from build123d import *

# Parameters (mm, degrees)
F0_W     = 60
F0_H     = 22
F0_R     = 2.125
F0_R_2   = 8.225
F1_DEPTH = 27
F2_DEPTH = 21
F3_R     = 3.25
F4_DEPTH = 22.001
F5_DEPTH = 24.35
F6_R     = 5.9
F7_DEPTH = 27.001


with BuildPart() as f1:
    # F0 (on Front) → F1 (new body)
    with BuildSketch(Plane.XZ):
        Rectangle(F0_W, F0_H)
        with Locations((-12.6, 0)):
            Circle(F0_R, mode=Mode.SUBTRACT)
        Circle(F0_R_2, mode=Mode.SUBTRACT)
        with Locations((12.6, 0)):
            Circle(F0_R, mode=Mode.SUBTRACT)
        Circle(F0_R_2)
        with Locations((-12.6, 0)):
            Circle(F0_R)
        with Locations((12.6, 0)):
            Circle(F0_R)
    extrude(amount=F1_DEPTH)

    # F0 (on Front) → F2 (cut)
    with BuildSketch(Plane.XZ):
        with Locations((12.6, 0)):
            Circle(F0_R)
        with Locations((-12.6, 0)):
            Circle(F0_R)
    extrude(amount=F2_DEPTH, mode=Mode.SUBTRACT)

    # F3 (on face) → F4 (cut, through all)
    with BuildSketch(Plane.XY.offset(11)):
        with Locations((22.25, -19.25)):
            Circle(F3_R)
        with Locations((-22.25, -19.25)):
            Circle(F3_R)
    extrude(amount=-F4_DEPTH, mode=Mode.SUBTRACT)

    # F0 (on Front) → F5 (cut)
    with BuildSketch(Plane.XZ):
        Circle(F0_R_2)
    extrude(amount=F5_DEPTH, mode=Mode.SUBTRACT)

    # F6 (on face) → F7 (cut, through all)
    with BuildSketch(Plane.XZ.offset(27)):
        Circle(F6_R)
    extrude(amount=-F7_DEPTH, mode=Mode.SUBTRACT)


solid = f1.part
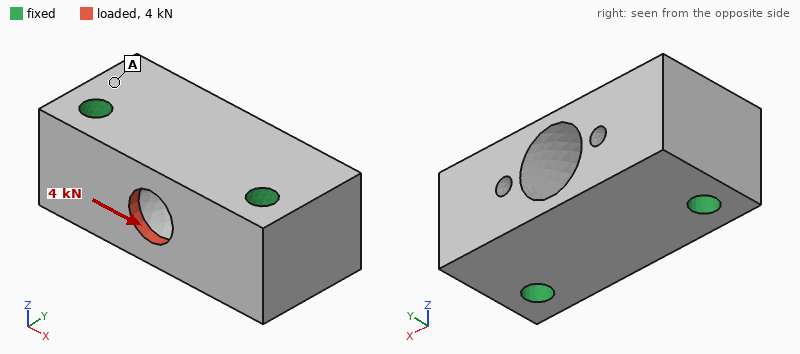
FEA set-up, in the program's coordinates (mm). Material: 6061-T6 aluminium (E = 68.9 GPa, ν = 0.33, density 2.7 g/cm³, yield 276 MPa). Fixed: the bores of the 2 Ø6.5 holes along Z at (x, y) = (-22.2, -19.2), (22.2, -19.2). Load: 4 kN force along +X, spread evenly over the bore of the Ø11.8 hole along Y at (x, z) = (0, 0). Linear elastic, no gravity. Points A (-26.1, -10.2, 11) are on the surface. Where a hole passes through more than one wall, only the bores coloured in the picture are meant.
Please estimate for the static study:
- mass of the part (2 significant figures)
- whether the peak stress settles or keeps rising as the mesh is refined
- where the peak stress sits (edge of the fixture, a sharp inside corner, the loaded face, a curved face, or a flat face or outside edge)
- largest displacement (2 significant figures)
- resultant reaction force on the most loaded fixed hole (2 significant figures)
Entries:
76 g
keeps rising
a sharp inside corner
6.6 µm
2.1 kN
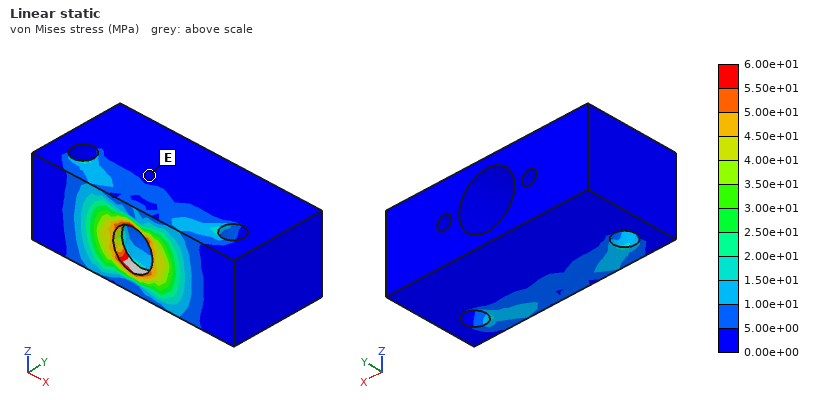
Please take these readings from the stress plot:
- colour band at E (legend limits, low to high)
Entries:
0.00e+00 to 5.00e+00 MPa
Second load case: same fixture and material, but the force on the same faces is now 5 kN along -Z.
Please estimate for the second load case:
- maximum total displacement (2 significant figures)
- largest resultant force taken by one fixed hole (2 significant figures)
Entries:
25 µm
2.5 kN
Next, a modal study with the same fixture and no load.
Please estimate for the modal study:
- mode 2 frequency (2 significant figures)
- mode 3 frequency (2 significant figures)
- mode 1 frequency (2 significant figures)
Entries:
24 kHz
29 kHz
24 kHz
